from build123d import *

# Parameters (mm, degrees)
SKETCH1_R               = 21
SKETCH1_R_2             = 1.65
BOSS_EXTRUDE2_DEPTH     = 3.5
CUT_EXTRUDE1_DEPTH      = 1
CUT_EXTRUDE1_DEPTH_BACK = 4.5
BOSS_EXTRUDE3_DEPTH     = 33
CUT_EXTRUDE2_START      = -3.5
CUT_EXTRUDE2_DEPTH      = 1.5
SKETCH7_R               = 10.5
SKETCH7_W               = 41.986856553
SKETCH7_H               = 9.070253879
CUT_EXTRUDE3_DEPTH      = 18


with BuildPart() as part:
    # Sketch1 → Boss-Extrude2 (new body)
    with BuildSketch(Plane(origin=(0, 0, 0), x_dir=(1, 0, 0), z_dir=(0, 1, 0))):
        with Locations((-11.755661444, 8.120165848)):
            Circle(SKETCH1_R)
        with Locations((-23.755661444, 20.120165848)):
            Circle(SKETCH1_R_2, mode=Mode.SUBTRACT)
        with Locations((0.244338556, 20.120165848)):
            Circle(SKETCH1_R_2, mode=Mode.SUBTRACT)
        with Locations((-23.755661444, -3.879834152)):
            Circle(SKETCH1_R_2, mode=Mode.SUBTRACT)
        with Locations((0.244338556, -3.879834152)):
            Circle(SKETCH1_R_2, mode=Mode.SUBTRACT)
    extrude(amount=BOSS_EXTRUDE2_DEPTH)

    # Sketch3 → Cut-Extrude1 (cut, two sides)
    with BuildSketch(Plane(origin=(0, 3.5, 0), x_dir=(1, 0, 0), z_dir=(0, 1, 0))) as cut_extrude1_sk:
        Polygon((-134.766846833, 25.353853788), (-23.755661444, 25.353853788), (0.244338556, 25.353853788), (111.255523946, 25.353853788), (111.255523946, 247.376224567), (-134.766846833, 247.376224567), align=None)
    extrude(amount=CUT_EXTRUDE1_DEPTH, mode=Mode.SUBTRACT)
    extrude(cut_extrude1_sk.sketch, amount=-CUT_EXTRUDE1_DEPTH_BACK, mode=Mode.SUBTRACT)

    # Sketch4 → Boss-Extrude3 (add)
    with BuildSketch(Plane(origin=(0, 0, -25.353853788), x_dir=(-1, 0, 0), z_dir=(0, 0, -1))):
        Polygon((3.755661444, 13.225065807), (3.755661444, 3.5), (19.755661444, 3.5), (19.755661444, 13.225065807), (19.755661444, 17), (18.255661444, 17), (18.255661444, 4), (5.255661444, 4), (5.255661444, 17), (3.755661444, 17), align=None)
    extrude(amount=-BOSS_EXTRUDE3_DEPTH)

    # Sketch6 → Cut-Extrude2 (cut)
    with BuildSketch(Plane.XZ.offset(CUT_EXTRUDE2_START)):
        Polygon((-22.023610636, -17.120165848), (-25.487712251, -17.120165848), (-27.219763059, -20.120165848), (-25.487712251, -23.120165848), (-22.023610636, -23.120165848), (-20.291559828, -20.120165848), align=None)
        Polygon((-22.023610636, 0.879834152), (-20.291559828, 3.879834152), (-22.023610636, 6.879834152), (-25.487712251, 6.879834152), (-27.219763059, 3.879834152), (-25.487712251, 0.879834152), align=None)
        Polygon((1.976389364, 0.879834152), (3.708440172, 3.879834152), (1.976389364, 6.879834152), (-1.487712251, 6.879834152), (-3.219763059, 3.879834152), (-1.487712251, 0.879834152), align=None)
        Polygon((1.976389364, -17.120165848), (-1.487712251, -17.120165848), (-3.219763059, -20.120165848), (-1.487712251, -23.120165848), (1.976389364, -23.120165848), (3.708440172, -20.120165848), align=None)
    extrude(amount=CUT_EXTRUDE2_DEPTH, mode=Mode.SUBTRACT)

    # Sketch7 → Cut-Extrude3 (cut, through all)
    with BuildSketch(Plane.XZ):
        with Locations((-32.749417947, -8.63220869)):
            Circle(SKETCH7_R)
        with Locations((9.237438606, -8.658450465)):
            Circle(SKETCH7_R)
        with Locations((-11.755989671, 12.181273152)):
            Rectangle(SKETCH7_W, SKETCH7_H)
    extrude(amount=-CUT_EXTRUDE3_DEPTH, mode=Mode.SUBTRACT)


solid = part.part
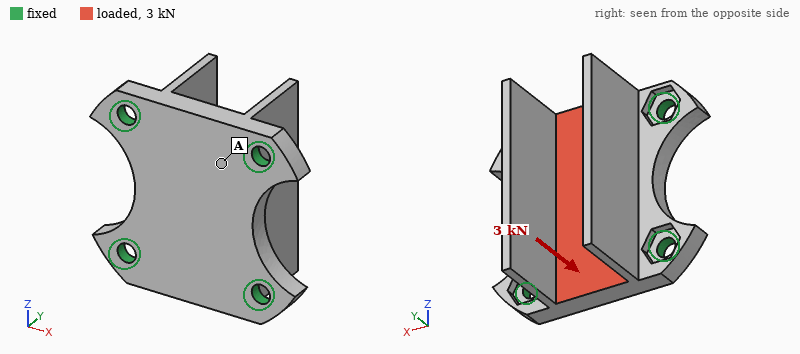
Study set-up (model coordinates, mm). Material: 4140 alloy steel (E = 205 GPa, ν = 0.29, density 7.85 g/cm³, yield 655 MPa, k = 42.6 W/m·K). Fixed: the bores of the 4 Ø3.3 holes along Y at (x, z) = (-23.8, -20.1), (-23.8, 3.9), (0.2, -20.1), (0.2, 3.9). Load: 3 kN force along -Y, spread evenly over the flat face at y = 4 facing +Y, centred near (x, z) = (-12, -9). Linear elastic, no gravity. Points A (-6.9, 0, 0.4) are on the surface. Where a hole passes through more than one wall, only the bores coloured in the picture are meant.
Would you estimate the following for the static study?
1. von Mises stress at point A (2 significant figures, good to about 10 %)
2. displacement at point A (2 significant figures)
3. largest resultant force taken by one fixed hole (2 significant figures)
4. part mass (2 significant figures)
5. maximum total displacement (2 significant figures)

39 MPa
8.5 µm
1.1 kN
35 g
18 µm
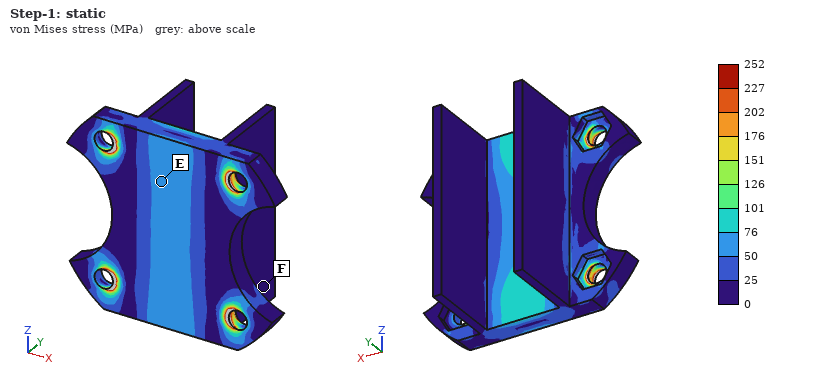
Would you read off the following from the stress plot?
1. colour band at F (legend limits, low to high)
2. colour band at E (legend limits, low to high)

0 to 25 MPa
50 to 76 MPa
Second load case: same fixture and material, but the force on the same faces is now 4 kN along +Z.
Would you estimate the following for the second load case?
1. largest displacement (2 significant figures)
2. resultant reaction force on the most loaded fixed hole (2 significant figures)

6.7 µm
1.1 kN
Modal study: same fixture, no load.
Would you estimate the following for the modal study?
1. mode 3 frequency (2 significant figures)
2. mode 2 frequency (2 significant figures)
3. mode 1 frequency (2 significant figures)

9000 Hz
6700 Hz
6500 Hz
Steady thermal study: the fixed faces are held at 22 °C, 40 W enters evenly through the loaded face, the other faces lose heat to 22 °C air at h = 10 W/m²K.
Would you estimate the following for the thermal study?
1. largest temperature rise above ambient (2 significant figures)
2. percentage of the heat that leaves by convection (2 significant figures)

60 K
3.3 %
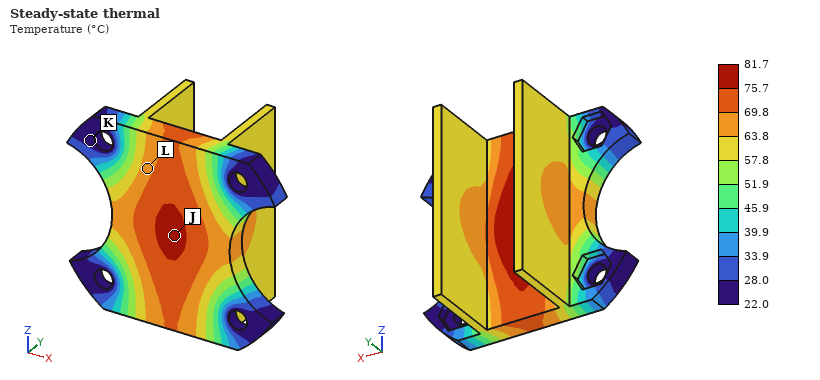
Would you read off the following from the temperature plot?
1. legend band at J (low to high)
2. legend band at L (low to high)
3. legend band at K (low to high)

75.7 to 81.7 °C
63.8 to 69.8 °C
22.0 to 28.0 °C
